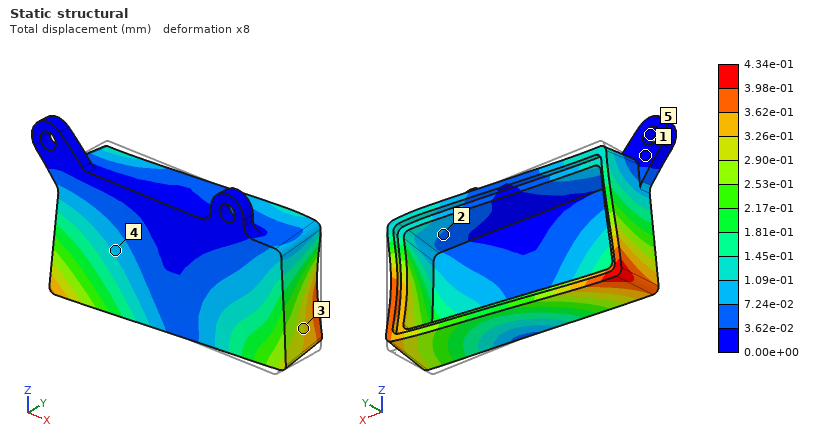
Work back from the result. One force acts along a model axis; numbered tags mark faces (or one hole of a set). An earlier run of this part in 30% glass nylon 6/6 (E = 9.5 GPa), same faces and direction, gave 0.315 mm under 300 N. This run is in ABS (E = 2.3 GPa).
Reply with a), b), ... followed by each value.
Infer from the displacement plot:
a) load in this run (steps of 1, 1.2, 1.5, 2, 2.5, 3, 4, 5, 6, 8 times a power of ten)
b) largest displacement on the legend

a) 100 N
b) 4.34e-01 mm
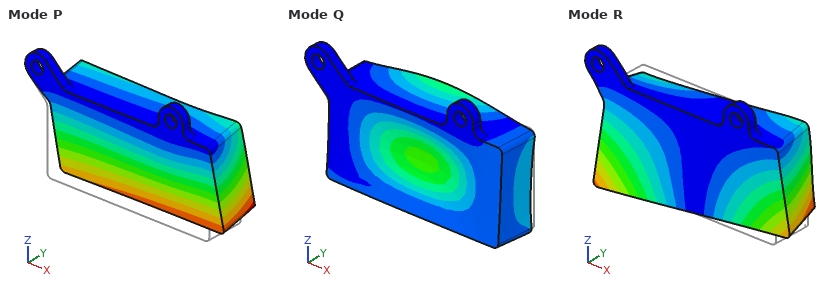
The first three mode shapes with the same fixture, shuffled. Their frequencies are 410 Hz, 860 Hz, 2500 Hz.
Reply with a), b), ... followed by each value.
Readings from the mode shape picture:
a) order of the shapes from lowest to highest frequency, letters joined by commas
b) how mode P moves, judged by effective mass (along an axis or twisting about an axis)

a) P, R, Q
b) along Y
